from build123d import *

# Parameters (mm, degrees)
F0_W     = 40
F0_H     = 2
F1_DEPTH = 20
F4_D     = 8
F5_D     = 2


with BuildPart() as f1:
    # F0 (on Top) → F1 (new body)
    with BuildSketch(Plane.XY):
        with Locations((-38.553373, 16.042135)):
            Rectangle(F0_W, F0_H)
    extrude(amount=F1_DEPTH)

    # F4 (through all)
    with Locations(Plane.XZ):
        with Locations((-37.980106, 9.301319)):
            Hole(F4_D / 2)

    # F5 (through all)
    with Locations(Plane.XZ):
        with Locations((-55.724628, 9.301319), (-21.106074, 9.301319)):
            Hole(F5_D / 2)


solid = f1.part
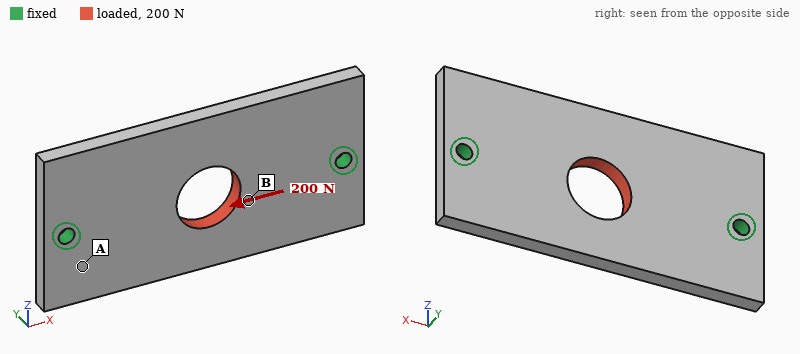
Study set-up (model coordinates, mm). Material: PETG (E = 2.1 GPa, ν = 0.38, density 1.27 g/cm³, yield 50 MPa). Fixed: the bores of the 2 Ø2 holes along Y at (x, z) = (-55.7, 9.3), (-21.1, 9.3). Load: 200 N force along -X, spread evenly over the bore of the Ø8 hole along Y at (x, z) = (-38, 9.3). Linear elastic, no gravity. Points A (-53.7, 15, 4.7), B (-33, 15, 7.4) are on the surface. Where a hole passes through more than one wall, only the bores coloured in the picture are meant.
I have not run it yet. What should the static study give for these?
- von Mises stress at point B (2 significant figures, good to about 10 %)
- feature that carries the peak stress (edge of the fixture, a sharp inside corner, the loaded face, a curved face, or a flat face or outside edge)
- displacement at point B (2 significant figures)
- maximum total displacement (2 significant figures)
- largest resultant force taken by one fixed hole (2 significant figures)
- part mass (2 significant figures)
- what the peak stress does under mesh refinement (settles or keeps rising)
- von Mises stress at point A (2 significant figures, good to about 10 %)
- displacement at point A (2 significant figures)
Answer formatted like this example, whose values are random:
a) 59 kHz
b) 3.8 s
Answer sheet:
a) 4.9 MPa
b) edge of the fixture
c) 33 µm
d) 41 µm
e) 100 N
f) 1.9 g
g) keeps rising
h) 2.1 MPa
i) 18 µm
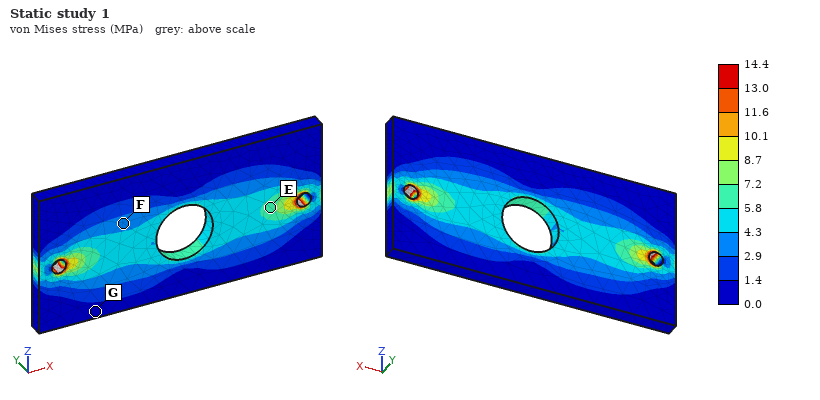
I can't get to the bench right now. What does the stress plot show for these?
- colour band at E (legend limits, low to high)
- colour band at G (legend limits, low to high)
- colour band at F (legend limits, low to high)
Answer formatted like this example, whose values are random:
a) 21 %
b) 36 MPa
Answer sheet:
a) 5.8 to 7.2 MPa
b) 0.0 to 1.4 MPa
c) 2.9 to 4.3 MPa
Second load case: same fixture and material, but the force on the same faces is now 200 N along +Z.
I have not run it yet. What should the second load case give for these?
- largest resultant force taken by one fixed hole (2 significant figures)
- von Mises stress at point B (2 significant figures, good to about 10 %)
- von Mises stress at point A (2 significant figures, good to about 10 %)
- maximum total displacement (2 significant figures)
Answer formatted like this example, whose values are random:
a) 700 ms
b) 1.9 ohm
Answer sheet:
a) 100 N
b) 6.4 MPa
c) 3.6 MPa
d) 0.12 mm
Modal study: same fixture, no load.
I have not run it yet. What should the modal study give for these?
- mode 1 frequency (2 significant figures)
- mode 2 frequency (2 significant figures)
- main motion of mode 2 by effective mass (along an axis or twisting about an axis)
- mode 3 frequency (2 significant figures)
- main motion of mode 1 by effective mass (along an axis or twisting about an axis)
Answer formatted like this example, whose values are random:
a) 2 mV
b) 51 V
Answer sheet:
a) 1700 Hz
b) 2000 Hz
c) along Y
d) 3500 Hz
e) along Y
